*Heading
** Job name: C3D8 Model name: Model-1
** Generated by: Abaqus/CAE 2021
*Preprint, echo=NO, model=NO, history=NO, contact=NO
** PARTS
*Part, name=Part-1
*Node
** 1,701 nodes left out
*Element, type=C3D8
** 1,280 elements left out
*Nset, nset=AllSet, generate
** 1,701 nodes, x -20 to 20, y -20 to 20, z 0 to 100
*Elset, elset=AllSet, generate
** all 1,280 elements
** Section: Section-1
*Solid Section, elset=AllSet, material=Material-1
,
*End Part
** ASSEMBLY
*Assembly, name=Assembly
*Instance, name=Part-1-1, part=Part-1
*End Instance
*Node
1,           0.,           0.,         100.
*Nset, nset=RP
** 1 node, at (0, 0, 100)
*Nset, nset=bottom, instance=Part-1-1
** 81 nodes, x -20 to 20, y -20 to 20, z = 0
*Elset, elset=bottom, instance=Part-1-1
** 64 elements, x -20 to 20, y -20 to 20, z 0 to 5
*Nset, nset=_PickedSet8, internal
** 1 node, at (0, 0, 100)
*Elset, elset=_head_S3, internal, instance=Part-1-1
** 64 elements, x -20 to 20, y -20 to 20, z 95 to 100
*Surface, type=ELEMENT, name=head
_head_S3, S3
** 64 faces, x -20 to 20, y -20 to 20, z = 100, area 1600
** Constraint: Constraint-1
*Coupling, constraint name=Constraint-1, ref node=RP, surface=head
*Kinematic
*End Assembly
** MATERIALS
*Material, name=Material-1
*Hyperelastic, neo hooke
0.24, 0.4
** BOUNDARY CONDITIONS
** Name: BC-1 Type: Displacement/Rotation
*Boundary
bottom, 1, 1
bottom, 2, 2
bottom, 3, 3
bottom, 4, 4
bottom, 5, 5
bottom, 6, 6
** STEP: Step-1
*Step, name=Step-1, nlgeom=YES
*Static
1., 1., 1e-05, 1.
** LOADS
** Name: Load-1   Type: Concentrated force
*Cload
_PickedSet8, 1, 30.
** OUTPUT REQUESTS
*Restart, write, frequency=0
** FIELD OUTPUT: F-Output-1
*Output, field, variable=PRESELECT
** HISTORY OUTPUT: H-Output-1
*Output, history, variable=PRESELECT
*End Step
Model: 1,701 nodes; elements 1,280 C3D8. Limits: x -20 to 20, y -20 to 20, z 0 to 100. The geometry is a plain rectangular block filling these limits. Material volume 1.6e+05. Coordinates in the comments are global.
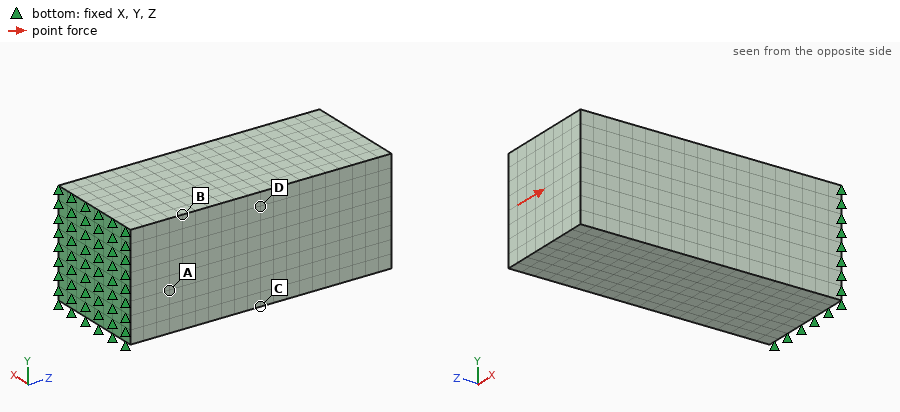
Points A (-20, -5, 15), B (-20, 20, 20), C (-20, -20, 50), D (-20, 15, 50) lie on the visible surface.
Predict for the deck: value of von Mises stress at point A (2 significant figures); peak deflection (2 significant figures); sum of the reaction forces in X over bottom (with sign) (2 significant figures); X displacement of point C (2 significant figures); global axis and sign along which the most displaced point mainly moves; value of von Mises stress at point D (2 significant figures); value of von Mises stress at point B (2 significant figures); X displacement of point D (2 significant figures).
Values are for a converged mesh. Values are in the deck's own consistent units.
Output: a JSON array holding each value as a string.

["0.23", "35", "-30", "12", "+X", "0.14", "0.21", "13"]
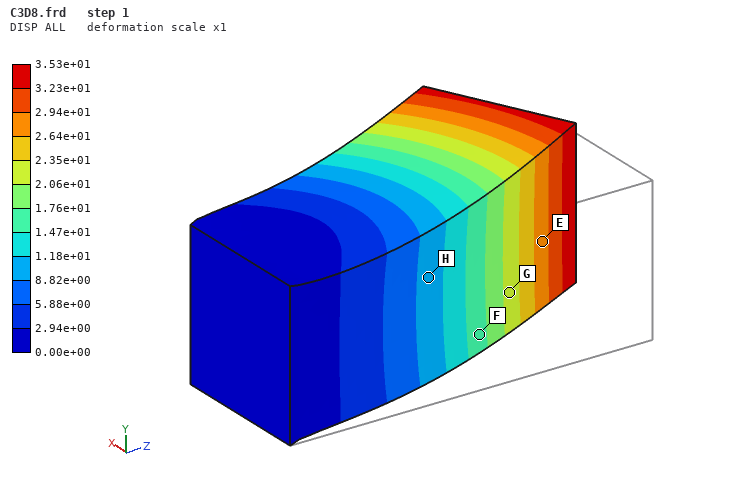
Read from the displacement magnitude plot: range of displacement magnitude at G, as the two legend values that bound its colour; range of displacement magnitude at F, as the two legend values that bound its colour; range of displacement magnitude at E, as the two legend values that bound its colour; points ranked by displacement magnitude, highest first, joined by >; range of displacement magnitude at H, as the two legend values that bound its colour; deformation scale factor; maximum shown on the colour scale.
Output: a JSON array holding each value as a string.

["2.06e+01 to 2.35e+01", "1.47e+01 to 1.76e+01", "2.64e+01 to 2.94e+01", "E > G > F > H", "8.82e+00 to 1.18e+01", "1", "3.53e+01"]
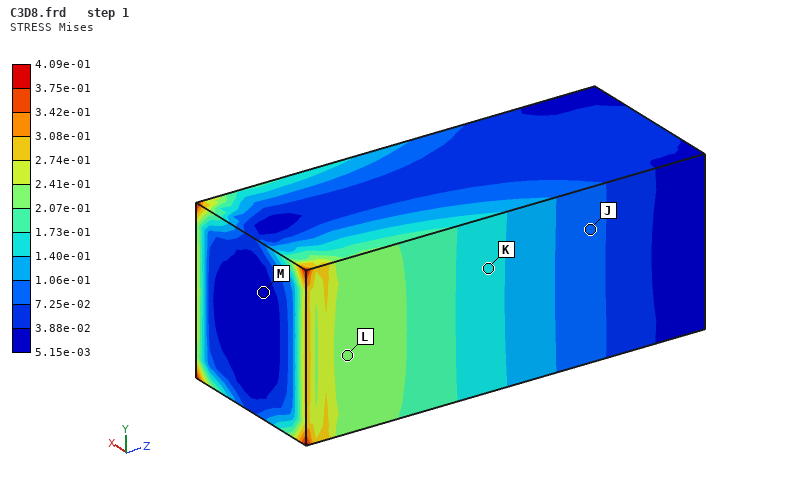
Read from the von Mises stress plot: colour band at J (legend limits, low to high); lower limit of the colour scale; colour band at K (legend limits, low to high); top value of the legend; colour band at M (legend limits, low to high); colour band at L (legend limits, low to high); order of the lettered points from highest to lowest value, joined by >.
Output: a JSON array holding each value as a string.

["7.25e-02 to 1.06e-01", "5.15e-03", "1.40e-01 to 1.73e-01", "4.09e-01", "5.15e-03 to 3.88e-02", "2.07e-01 to 2.41e-01", "L > K > J > M"]
